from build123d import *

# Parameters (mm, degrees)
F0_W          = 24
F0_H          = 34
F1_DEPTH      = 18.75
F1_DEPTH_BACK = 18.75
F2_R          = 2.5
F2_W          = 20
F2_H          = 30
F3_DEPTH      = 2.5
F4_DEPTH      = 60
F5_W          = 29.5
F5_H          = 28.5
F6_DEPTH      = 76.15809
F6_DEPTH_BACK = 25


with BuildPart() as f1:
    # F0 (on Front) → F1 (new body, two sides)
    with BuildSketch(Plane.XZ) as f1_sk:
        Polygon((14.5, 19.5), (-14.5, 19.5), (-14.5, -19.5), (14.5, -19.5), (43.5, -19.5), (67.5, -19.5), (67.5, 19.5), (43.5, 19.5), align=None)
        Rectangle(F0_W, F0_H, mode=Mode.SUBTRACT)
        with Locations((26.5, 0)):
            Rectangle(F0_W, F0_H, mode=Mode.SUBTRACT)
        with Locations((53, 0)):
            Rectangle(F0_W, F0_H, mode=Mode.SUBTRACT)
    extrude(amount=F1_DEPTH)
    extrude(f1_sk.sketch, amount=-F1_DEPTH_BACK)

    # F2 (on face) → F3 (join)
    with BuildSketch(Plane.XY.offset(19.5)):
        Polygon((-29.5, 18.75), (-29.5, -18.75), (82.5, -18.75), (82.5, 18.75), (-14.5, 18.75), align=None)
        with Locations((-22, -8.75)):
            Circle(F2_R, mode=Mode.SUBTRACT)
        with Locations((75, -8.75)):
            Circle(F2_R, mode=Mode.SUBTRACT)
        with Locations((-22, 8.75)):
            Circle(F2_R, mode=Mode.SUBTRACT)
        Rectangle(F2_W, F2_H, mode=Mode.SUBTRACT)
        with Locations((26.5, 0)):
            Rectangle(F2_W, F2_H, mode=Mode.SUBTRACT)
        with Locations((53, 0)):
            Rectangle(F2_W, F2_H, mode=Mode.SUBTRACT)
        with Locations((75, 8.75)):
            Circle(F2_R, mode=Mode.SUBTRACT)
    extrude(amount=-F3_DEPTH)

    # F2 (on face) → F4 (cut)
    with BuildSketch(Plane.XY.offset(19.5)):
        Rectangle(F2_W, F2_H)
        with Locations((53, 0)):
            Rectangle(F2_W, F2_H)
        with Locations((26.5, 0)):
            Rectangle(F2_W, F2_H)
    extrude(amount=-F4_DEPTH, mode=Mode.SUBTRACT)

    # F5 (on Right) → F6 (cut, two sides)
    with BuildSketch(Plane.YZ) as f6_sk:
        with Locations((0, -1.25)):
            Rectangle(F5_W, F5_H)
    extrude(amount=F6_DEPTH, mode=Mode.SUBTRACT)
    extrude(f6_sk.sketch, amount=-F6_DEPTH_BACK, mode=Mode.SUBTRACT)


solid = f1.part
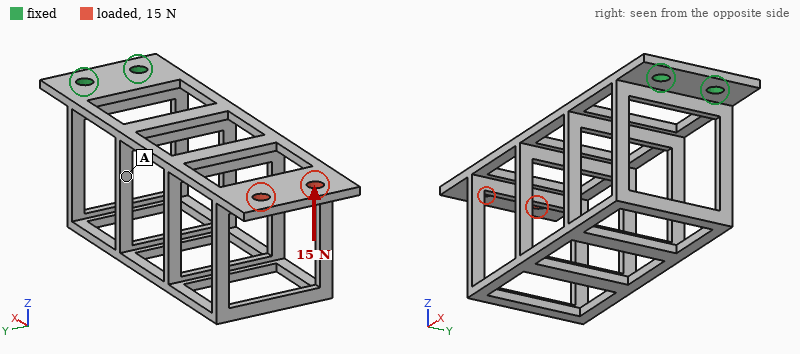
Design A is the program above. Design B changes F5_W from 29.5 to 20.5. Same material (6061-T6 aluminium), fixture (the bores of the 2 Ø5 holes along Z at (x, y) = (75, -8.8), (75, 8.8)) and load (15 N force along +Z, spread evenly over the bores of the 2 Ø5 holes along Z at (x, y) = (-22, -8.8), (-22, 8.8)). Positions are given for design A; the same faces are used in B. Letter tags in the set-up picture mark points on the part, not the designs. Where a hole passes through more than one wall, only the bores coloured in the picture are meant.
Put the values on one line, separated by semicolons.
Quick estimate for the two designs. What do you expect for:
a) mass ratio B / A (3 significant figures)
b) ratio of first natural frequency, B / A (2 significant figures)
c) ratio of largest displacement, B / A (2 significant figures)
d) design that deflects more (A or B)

1.19; 1.1; 0.76; A
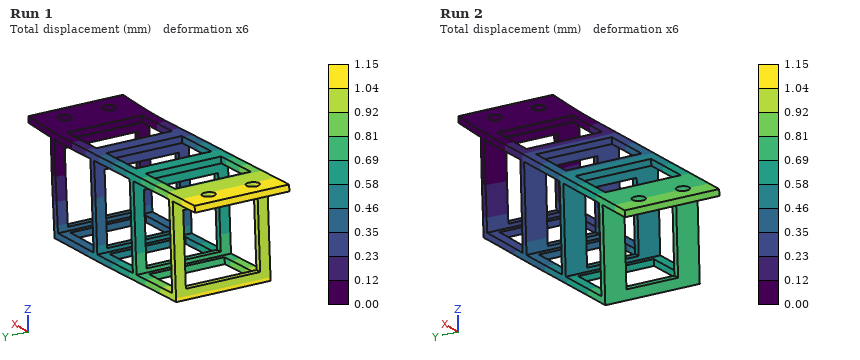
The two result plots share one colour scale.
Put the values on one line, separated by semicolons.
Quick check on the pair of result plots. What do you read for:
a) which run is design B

Run 2
